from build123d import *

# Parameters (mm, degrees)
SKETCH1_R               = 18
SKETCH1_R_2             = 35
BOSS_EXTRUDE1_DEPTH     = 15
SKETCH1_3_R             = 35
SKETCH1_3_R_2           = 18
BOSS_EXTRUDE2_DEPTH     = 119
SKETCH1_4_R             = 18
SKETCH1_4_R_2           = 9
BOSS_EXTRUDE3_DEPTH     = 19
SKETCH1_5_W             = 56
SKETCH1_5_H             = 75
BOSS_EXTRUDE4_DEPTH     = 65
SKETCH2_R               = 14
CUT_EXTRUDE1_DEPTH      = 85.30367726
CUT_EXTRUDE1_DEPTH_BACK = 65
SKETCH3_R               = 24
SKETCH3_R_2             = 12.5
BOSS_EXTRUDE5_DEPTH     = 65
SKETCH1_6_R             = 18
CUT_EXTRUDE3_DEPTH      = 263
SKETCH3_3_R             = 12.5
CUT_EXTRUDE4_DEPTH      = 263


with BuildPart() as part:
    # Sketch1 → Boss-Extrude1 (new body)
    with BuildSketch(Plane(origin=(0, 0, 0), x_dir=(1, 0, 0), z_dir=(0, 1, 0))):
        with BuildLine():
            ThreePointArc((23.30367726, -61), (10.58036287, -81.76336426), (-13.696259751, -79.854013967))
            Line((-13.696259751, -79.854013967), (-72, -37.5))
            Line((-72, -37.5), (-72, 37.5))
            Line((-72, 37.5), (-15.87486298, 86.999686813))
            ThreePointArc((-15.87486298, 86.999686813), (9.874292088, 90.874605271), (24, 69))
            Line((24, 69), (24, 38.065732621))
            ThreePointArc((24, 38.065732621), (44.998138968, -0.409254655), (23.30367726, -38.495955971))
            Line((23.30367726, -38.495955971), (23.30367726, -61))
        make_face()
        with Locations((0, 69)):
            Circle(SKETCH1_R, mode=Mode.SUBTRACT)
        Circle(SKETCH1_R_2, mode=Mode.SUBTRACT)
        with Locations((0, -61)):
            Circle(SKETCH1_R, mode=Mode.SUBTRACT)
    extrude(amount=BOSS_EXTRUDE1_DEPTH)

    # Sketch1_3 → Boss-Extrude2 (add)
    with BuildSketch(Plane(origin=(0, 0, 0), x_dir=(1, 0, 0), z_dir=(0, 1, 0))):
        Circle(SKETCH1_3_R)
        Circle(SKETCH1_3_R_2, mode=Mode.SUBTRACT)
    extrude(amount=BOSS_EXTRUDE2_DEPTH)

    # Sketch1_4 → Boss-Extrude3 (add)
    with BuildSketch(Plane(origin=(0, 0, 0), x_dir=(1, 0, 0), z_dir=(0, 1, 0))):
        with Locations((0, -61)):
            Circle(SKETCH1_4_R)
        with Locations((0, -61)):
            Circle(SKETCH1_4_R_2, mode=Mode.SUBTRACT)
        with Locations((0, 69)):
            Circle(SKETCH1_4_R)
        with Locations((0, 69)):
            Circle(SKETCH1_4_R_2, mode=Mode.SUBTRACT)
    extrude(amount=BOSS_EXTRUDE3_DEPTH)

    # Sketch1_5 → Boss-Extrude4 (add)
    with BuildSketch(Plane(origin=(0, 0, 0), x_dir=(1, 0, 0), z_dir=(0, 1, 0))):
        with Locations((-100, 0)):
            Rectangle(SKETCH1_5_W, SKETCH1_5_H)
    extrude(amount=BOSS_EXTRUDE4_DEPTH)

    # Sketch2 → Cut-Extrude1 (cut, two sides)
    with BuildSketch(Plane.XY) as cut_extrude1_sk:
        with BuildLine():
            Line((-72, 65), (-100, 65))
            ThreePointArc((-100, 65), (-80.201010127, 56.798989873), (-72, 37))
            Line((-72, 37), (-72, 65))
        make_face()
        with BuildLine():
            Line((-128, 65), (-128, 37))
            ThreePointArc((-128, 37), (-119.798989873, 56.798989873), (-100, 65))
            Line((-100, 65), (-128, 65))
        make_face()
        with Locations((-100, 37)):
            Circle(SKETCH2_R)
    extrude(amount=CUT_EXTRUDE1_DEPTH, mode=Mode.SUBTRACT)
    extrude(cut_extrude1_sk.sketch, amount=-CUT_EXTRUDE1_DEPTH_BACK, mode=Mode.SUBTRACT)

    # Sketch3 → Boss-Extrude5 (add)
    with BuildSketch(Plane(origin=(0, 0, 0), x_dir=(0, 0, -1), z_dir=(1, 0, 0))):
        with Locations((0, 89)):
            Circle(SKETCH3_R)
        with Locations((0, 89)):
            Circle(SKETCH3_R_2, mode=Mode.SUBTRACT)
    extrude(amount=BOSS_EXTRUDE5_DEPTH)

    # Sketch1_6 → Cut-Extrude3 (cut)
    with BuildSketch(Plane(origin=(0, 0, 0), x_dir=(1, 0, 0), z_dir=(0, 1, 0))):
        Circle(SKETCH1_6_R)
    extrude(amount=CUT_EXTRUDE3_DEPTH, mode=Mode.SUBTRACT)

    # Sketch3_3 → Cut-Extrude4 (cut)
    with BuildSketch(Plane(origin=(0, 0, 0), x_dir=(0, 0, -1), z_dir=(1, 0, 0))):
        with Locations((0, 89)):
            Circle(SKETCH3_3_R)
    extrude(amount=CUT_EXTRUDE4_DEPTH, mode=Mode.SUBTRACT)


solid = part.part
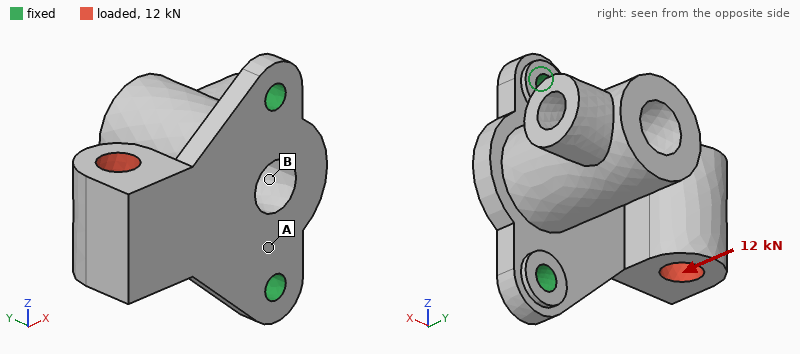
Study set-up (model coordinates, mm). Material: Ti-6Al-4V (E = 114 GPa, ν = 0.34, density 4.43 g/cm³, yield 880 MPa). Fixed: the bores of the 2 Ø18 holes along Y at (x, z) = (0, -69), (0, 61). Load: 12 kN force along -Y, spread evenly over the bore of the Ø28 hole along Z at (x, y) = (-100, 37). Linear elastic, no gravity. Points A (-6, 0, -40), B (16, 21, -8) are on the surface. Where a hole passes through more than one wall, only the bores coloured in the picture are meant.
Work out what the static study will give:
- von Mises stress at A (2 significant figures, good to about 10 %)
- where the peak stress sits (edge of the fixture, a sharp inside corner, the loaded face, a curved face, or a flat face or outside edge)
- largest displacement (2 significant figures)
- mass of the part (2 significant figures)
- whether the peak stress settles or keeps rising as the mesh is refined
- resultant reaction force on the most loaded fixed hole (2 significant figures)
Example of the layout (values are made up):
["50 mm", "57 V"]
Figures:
["91 MPa", "edge of the fixture", "1.4 mm", "3.2 kg", "keeps rising", "6.6 kN"]
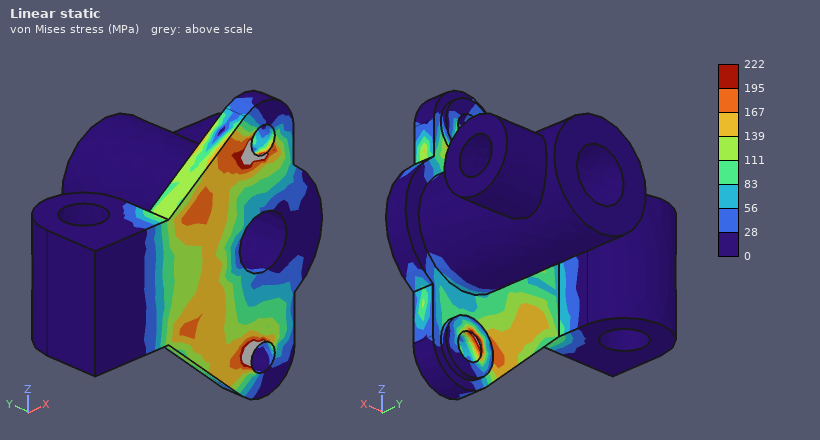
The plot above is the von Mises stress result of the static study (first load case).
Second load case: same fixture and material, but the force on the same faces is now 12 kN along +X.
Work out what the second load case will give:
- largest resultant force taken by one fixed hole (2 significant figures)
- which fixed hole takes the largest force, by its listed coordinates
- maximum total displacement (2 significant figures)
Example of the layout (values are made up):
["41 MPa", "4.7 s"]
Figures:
["6.8 kN", "(0, 61)", "0.67 mm"]
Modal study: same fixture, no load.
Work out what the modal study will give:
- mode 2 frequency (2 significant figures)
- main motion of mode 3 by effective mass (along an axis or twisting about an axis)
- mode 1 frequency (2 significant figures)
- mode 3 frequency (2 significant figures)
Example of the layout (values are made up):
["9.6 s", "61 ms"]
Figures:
["1100 Hz", "along Z", "500 Hz", "1700 Hz"]
